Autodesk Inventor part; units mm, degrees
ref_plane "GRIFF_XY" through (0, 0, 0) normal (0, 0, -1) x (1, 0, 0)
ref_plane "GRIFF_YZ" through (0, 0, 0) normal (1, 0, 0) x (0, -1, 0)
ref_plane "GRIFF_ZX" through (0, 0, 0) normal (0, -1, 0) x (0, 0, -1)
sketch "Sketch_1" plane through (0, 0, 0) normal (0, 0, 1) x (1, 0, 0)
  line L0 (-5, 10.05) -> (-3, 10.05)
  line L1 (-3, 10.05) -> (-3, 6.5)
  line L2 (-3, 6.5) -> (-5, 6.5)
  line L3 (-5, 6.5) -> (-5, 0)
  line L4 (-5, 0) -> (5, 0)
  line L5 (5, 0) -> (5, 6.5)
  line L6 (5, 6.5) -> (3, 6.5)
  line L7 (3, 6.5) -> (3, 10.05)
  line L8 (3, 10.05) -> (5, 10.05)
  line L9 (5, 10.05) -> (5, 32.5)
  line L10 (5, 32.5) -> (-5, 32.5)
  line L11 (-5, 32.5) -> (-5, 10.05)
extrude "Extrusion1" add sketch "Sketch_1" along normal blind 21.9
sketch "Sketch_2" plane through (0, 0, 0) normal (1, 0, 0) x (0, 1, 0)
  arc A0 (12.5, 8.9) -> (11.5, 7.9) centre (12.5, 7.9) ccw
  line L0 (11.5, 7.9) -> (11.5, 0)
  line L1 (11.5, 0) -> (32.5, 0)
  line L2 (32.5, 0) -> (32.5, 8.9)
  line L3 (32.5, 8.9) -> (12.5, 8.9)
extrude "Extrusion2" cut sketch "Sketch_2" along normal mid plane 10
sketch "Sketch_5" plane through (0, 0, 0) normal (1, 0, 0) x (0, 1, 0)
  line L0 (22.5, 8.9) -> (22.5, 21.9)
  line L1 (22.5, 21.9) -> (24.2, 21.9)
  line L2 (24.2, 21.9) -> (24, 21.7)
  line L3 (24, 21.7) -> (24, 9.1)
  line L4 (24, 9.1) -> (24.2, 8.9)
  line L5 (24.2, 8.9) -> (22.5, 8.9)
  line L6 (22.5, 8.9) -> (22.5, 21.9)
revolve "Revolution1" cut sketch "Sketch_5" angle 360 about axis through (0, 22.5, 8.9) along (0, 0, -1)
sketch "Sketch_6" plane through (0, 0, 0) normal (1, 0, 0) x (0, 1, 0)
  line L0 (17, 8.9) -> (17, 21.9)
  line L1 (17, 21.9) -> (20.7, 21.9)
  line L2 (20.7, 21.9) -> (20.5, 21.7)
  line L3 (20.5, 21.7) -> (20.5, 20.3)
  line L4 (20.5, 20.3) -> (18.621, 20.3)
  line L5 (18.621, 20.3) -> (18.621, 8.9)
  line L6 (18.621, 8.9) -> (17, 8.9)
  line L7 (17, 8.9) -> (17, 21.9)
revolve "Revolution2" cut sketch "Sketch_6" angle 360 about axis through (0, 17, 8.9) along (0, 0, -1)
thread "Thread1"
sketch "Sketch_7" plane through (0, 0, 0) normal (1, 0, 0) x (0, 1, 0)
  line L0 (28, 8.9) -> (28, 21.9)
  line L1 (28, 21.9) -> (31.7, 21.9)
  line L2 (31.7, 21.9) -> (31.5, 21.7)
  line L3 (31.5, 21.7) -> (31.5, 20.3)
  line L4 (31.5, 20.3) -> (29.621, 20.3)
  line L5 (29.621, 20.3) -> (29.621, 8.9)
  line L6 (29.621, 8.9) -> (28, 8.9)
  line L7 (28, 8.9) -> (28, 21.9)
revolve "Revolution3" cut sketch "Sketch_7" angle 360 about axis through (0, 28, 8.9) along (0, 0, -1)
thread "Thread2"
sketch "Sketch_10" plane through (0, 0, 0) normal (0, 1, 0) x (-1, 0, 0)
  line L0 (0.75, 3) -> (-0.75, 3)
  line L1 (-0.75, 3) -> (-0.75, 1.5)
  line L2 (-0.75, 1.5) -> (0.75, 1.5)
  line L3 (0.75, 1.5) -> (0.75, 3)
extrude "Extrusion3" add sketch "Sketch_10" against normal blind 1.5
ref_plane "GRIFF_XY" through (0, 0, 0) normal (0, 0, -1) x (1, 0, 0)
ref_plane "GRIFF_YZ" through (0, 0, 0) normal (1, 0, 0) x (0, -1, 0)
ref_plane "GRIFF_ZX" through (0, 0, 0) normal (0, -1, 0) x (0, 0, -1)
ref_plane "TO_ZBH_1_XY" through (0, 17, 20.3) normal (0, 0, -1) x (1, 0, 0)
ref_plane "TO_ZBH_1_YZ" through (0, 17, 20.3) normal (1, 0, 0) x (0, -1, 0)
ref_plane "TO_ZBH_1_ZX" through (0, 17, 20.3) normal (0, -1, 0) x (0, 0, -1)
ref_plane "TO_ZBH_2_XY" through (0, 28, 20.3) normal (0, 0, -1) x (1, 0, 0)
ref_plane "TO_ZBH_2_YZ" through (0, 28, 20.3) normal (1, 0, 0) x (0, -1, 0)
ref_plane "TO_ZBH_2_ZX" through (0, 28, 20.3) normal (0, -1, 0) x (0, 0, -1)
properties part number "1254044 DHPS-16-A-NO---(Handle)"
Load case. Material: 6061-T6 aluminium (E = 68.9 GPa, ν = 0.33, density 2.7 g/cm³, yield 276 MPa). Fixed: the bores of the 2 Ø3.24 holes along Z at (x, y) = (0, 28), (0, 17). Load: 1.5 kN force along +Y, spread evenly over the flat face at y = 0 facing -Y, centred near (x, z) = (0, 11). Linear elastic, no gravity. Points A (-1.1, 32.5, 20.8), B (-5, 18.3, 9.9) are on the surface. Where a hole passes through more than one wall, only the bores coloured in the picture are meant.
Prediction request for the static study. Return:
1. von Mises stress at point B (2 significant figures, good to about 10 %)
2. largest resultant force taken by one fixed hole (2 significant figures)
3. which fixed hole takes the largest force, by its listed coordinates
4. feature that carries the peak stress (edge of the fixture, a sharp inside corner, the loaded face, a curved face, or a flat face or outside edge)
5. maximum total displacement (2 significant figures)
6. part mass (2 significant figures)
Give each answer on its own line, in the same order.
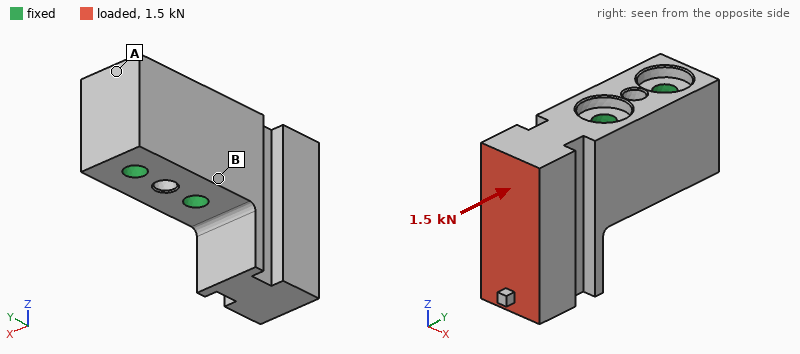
16 MPa
1.4 kN
(0, 17)
a curved face
18 µm
12 g
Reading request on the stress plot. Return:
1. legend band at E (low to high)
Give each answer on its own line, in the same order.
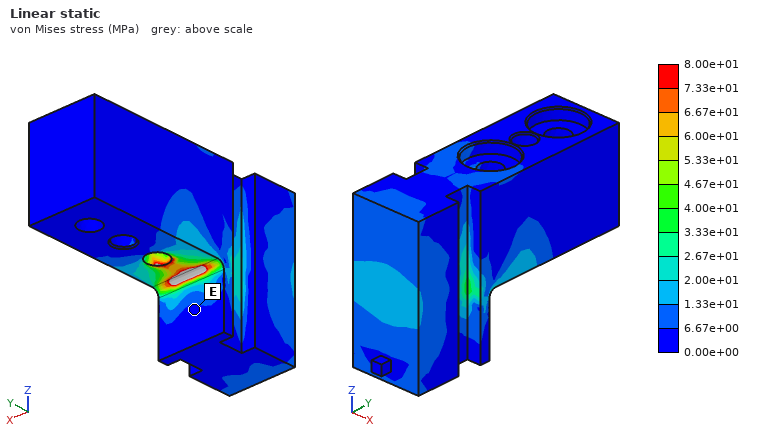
0.00e+00 to 6.67e+00 MPa
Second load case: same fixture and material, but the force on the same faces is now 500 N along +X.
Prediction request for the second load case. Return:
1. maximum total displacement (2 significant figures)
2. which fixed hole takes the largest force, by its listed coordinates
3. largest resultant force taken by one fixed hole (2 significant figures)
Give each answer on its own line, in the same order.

38 µm
(0, 17)
830 N
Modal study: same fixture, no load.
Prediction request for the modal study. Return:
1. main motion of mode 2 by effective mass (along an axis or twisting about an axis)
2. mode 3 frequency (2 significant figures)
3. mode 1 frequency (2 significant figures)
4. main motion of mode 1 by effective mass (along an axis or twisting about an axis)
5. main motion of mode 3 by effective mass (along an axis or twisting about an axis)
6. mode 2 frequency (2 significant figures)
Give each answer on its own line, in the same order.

along Z
21 kHz
12 kHz
along X
twisting about Y
16 kHz
